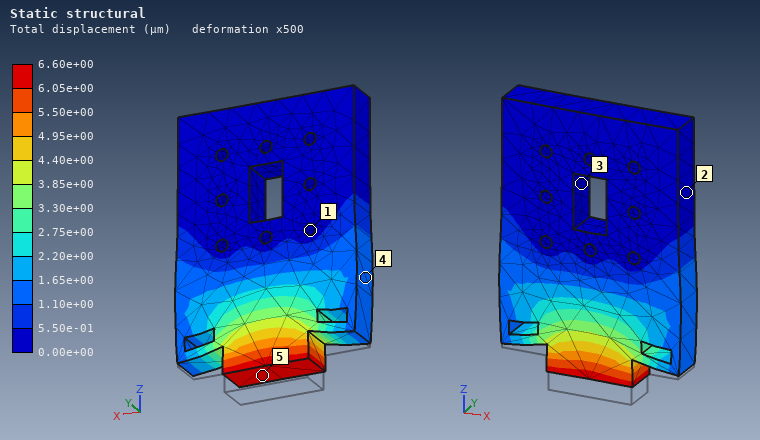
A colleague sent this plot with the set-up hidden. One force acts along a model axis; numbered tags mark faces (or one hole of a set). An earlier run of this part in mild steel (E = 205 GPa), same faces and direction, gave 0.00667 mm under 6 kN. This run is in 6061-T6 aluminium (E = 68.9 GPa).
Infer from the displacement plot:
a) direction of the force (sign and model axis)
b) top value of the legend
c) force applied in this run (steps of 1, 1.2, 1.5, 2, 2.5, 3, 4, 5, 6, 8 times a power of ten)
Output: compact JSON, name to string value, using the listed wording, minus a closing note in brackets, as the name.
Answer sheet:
{"direction of the force": "+Z", "top value of the legend": "6.60e+00 µm", "force applied in this run": "2 kN"}
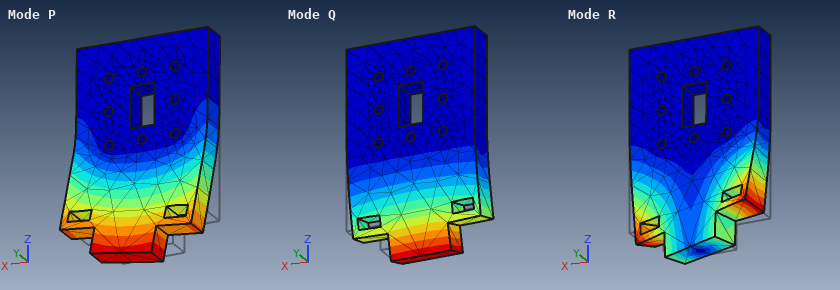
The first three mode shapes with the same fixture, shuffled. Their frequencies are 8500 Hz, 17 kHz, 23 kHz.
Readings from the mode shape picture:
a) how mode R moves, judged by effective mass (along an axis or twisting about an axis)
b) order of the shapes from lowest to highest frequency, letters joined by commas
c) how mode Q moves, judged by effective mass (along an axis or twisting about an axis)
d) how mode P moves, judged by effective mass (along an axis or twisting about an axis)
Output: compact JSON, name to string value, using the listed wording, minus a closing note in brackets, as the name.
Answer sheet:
{"how mode R moves, judged by effective mass": "twisting about Z", "order of the shapes from lowest to highest frequency, letters joined by commas": "Q, R, P", "how mode Q moves, judged by effective mass": "along Y", "how mode P moves, judged by effective mass": "along X"}
